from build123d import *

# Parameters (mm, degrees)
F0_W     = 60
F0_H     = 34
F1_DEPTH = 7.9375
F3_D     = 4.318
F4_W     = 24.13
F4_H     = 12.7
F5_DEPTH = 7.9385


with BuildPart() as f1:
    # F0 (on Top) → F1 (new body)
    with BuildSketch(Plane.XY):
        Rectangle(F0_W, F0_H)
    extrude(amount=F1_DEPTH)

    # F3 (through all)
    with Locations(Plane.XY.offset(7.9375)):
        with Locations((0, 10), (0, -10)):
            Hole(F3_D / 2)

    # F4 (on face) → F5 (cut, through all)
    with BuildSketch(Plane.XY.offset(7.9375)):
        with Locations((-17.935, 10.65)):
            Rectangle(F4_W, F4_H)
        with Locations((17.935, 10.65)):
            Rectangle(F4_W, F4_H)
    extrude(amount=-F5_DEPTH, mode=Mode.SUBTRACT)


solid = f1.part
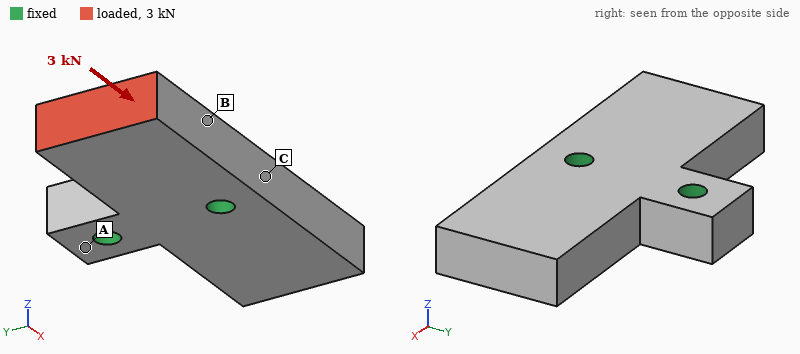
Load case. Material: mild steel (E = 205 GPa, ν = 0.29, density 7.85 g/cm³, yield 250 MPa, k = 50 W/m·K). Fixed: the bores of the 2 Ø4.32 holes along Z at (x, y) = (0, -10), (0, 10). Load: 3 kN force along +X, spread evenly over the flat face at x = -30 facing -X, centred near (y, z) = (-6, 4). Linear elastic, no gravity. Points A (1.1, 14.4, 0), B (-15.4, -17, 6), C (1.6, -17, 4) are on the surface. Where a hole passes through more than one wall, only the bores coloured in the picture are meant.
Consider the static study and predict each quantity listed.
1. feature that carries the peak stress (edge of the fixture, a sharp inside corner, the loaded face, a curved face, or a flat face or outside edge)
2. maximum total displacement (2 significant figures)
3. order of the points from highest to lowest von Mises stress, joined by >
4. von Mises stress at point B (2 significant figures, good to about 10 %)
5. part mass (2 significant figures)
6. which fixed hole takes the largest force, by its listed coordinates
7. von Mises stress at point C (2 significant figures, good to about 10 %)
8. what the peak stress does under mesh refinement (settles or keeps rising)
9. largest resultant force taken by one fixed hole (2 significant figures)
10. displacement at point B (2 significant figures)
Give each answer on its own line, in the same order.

edge of the fixture
3.0 µm
B > C > A
17 MPa
87 g
(0, -10)
9.9 MPa
keeps rising
2.4 kN
1.4 µm
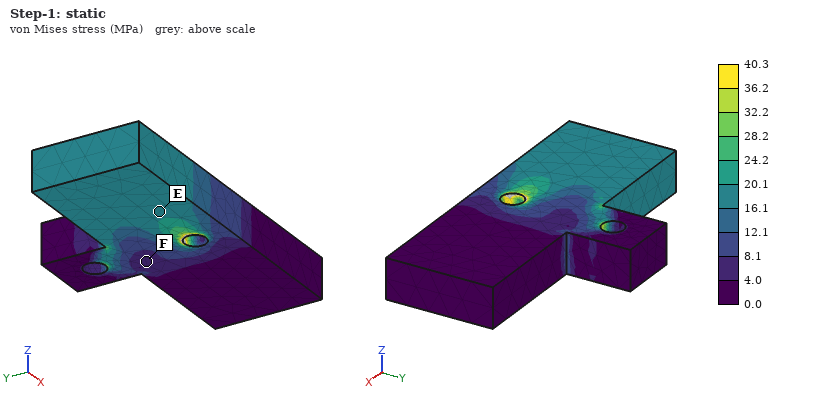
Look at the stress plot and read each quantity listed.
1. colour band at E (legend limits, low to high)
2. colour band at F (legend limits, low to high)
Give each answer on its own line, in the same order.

16.1 to 20.1 MPa
4.0 to 8.1 MPa
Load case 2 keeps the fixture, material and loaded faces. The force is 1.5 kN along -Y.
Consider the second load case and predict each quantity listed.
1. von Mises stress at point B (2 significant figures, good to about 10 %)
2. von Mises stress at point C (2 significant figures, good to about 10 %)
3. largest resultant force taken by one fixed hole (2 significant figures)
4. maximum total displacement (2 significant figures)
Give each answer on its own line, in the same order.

37 MPa
27 MPa
2.2 kN
18 µm
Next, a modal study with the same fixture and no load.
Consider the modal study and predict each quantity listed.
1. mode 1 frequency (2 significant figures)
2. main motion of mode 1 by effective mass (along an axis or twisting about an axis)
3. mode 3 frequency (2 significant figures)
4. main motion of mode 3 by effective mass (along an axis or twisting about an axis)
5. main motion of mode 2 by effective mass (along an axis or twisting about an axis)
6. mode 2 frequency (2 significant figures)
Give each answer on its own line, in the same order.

6400 Hz
twisting about Y
13 kHz
twisting about Z
along Z
7400 Hz
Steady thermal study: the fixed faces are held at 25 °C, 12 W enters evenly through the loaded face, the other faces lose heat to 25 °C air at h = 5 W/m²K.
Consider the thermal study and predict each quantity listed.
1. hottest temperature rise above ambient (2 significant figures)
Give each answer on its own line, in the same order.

42 K
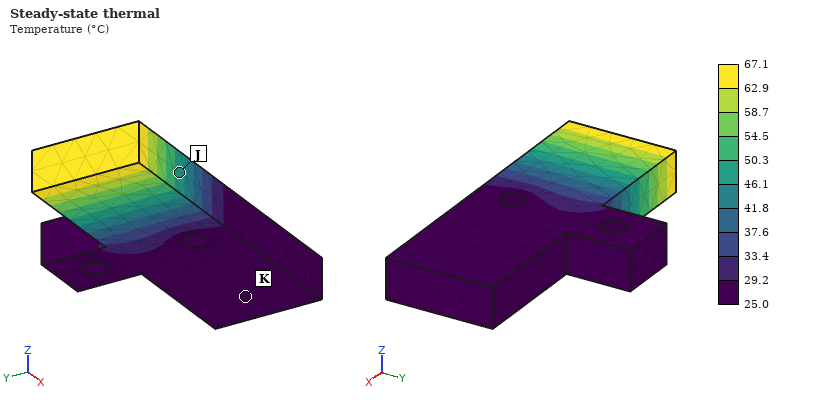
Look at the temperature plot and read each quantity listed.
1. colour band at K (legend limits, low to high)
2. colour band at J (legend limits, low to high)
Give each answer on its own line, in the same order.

25.0 to 29.2 °C
46.1 to 50.3 °C
